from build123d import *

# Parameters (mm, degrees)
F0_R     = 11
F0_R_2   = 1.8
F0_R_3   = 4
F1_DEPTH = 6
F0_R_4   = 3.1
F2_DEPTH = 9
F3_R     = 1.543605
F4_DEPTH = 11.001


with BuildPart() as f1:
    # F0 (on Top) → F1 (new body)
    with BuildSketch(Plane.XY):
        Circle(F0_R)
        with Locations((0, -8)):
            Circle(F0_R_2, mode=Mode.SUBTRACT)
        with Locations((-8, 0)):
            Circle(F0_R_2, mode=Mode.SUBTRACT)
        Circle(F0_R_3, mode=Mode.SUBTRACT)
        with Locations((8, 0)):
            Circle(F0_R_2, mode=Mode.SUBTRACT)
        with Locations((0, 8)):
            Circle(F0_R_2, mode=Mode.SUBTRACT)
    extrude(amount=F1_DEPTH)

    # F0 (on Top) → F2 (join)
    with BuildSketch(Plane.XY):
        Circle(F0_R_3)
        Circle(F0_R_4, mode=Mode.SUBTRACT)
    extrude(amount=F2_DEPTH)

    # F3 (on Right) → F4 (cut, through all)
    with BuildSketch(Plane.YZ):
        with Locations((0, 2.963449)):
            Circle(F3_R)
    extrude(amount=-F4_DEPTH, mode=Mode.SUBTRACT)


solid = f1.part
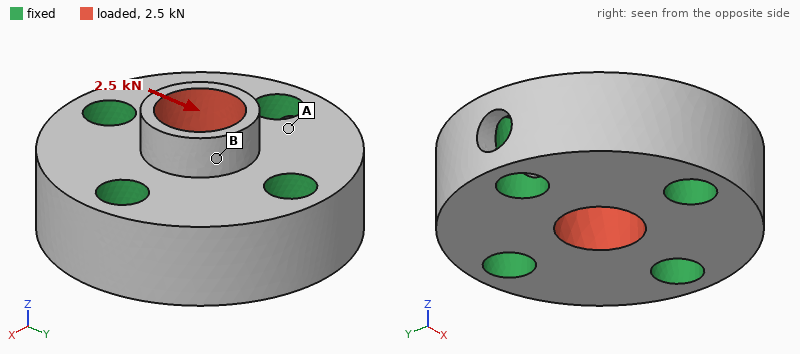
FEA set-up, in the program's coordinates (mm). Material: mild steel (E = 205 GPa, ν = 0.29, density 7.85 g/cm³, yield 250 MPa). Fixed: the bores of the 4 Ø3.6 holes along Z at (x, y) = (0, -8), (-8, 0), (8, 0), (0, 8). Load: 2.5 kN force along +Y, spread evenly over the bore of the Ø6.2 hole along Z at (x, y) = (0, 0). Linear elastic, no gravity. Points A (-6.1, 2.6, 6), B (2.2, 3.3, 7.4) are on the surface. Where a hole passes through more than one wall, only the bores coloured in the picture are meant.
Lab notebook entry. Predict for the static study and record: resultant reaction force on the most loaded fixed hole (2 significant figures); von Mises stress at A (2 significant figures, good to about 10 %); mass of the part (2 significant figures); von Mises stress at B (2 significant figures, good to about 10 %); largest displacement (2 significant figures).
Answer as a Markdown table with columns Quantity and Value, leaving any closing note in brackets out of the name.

| Quantity | Value |
|---|---|
| resultant reaction force on the most loaded fixed hole | 860 N |
| von Mises stress at A | 12 MPa |
| mass of the part | 15 g |
| von Mises stress at B | 37 MPa |
| largest displacement | 4.0 µm |
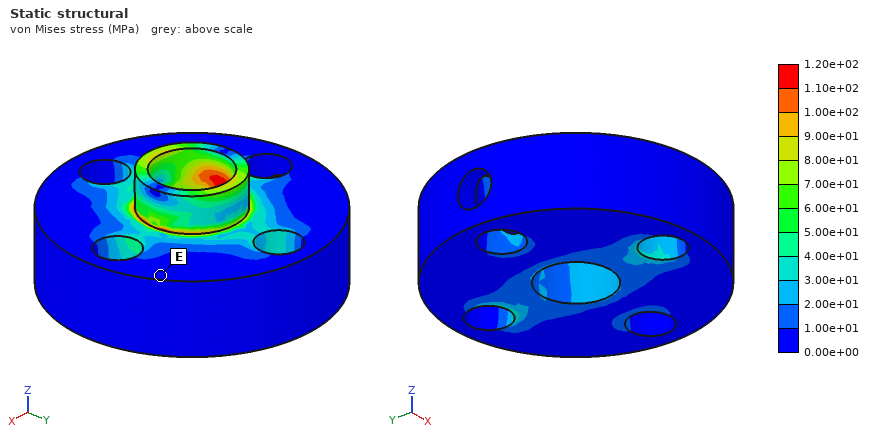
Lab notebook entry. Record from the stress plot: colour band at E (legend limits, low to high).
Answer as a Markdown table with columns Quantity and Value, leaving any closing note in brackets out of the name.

| Quantity | Value |
|---|---|
| colour band at E | 0.00e+00 to 1.00e+01 MPa |
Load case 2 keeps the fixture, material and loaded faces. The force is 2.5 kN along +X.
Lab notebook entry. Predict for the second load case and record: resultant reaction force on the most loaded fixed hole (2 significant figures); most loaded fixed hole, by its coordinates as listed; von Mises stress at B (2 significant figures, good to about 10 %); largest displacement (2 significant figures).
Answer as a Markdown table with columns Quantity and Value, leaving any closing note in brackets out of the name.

| Quantity | Value |
|---|---|
| resultant reaction force on the most loaded fixed hole | 870 N |
| most loaded fixed hole, by its coordinates as listed | (8, 0) |
| von Mises stress at B | 47 MPa |
| largest displacement | 4.1 µm |
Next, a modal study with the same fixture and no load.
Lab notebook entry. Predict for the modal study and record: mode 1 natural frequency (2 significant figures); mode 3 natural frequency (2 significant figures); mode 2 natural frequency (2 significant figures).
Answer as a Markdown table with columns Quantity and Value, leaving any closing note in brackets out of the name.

| Quantity | Value |
|---|---|
| mode 1 natural frequency | 110 kHz |
| mode 3 natural frequency | 120 kHz |
| mode 2 natural frequency | 120 kHz |
